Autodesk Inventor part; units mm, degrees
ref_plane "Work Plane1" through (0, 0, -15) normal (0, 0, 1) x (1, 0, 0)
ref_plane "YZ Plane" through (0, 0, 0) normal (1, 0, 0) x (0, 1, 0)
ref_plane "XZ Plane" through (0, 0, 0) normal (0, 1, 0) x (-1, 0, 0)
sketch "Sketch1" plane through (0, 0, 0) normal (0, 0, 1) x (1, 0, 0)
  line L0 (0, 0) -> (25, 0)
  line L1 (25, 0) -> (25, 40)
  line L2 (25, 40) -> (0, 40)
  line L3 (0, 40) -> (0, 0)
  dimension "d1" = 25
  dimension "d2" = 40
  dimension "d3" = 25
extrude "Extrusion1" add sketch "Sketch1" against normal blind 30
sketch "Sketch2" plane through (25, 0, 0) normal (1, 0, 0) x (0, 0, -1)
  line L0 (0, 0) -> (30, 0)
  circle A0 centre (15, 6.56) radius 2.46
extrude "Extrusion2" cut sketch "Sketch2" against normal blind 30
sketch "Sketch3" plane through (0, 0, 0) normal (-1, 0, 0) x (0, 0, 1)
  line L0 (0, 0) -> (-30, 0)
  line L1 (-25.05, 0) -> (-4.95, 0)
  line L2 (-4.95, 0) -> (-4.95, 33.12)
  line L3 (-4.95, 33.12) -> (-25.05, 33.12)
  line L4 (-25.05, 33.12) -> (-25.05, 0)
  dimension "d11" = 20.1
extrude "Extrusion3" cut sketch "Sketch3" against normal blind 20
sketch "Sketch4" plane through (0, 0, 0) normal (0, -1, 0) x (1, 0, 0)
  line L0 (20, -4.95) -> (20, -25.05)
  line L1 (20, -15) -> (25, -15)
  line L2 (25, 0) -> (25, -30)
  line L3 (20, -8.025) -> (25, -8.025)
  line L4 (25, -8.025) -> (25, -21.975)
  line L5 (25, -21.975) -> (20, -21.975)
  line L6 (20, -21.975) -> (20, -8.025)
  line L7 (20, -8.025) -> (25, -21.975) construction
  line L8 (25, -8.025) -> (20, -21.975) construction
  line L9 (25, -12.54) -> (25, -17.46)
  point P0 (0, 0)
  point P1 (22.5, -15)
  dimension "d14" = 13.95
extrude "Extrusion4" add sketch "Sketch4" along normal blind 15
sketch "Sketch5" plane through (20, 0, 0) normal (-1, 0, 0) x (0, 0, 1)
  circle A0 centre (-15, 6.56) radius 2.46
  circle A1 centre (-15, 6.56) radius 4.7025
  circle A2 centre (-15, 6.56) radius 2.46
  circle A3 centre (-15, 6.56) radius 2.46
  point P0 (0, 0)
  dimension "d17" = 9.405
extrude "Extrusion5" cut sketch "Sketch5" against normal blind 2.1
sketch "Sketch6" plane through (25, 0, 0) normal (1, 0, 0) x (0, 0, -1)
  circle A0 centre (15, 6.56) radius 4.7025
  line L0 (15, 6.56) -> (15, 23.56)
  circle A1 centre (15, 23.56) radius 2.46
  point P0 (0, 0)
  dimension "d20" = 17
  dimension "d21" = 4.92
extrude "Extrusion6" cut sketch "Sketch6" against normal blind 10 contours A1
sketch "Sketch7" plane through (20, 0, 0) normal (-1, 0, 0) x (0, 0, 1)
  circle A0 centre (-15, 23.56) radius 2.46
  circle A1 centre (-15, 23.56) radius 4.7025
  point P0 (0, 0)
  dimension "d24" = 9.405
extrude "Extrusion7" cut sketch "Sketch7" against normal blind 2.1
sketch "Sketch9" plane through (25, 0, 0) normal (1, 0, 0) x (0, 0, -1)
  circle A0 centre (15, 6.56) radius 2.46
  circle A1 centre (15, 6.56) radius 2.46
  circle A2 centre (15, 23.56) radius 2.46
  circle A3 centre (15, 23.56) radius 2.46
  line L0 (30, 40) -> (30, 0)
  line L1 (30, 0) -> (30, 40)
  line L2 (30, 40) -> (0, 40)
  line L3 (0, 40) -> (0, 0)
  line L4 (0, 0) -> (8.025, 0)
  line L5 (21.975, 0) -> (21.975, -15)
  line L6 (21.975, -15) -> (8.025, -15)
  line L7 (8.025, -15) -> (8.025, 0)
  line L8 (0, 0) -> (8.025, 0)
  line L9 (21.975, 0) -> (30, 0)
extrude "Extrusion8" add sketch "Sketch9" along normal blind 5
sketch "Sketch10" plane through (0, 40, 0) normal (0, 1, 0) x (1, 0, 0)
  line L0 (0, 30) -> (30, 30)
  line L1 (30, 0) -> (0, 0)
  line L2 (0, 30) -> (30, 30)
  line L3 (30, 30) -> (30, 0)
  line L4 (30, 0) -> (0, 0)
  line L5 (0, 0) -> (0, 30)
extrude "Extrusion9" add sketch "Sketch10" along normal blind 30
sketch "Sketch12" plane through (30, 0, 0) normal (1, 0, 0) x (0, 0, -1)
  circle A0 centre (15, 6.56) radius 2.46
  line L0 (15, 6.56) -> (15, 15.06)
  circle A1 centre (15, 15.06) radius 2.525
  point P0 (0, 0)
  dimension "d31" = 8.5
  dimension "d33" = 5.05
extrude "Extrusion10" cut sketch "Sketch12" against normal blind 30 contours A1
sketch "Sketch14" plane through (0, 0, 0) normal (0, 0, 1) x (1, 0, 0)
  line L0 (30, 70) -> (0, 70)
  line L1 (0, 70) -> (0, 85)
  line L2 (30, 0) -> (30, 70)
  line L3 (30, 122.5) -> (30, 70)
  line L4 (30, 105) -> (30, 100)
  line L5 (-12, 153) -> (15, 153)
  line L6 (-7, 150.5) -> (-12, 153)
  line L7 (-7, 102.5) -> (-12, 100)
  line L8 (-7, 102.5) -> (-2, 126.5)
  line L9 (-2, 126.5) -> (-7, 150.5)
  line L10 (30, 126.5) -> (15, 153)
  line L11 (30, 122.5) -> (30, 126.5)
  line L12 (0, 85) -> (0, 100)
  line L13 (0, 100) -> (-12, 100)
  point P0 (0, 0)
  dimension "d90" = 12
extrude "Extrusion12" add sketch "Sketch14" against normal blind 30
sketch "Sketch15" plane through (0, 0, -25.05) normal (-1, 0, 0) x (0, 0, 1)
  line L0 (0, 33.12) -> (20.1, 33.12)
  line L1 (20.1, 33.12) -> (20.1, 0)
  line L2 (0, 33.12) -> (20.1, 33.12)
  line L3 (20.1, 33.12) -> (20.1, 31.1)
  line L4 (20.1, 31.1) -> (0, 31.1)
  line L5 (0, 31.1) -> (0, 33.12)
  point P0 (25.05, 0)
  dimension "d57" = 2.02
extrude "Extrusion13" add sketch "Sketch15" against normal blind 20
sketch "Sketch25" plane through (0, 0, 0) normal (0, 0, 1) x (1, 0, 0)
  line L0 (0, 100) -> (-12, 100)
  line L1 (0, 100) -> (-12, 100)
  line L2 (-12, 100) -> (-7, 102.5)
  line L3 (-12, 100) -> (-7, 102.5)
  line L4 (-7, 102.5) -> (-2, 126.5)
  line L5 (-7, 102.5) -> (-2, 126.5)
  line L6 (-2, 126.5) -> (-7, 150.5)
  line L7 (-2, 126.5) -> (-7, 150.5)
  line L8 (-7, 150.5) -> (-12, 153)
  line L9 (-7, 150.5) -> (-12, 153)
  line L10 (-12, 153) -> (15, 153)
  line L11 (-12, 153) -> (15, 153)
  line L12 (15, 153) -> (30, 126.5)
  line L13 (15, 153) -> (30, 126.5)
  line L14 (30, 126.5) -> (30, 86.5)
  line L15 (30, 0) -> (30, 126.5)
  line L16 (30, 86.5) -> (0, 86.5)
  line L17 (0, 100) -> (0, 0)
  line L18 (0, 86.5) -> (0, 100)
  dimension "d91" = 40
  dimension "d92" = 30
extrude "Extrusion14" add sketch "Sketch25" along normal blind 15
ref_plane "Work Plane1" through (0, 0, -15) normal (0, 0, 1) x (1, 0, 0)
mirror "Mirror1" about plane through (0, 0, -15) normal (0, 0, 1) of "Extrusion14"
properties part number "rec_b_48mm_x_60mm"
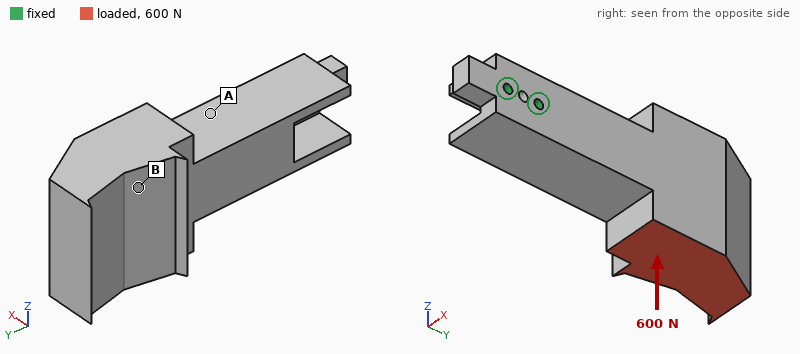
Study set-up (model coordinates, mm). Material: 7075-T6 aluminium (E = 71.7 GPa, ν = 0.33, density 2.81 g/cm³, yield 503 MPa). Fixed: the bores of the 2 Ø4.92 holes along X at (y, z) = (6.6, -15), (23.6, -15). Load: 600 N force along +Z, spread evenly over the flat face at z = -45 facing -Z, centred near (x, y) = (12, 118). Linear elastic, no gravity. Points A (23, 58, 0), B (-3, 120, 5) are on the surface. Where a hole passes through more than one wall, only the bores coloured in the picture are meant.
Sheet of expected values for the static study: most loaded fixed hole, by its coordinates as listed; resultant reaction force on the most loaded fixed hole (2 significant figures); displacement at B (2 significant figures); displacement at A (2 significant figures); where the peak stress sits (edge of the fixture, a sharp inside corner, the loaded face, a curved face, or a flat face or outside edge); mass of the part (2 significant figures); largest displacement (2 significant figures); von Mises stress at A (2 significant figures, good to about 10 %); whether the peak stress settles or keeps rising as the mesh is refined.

(23.6, -15)
3.0 kN
0.11 mm
0.036 mm
edge of the fixture
530 g
0.16 mm
8.6 MPa
keeps rising
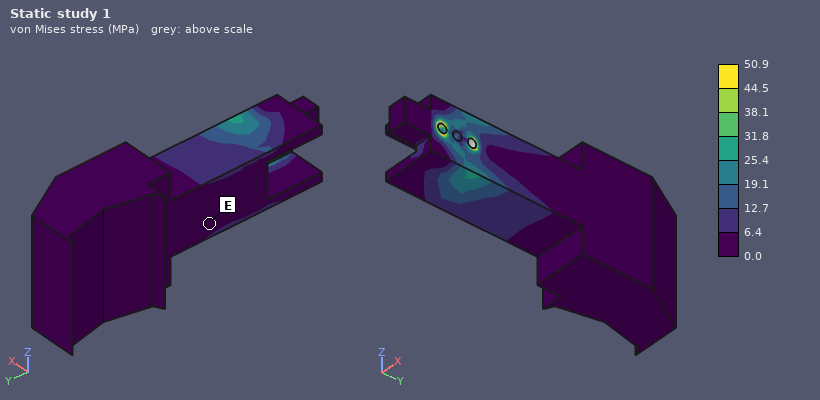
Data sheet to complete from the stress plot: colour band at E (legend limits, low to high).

0.0 to 6.4 MPa
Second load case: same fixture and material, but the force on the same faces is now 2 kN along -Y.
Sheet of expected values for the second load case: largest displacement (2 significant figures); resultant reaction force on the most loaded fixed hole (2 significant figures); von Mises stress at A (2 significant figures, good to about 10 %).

0.22 mm
3.1 kN
13 MPa
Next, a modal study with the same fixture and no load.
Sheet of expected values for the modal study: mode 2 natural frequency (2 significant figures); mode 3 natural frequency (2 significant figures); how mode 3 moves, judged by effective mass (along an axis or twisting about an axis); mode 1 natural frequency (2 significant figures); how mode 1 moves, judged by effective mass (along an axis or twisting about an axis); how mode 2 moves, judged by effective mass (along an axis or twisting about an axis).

590 Hz
1600 Hz
twisting about Y
520 Hz
along X
along Z
